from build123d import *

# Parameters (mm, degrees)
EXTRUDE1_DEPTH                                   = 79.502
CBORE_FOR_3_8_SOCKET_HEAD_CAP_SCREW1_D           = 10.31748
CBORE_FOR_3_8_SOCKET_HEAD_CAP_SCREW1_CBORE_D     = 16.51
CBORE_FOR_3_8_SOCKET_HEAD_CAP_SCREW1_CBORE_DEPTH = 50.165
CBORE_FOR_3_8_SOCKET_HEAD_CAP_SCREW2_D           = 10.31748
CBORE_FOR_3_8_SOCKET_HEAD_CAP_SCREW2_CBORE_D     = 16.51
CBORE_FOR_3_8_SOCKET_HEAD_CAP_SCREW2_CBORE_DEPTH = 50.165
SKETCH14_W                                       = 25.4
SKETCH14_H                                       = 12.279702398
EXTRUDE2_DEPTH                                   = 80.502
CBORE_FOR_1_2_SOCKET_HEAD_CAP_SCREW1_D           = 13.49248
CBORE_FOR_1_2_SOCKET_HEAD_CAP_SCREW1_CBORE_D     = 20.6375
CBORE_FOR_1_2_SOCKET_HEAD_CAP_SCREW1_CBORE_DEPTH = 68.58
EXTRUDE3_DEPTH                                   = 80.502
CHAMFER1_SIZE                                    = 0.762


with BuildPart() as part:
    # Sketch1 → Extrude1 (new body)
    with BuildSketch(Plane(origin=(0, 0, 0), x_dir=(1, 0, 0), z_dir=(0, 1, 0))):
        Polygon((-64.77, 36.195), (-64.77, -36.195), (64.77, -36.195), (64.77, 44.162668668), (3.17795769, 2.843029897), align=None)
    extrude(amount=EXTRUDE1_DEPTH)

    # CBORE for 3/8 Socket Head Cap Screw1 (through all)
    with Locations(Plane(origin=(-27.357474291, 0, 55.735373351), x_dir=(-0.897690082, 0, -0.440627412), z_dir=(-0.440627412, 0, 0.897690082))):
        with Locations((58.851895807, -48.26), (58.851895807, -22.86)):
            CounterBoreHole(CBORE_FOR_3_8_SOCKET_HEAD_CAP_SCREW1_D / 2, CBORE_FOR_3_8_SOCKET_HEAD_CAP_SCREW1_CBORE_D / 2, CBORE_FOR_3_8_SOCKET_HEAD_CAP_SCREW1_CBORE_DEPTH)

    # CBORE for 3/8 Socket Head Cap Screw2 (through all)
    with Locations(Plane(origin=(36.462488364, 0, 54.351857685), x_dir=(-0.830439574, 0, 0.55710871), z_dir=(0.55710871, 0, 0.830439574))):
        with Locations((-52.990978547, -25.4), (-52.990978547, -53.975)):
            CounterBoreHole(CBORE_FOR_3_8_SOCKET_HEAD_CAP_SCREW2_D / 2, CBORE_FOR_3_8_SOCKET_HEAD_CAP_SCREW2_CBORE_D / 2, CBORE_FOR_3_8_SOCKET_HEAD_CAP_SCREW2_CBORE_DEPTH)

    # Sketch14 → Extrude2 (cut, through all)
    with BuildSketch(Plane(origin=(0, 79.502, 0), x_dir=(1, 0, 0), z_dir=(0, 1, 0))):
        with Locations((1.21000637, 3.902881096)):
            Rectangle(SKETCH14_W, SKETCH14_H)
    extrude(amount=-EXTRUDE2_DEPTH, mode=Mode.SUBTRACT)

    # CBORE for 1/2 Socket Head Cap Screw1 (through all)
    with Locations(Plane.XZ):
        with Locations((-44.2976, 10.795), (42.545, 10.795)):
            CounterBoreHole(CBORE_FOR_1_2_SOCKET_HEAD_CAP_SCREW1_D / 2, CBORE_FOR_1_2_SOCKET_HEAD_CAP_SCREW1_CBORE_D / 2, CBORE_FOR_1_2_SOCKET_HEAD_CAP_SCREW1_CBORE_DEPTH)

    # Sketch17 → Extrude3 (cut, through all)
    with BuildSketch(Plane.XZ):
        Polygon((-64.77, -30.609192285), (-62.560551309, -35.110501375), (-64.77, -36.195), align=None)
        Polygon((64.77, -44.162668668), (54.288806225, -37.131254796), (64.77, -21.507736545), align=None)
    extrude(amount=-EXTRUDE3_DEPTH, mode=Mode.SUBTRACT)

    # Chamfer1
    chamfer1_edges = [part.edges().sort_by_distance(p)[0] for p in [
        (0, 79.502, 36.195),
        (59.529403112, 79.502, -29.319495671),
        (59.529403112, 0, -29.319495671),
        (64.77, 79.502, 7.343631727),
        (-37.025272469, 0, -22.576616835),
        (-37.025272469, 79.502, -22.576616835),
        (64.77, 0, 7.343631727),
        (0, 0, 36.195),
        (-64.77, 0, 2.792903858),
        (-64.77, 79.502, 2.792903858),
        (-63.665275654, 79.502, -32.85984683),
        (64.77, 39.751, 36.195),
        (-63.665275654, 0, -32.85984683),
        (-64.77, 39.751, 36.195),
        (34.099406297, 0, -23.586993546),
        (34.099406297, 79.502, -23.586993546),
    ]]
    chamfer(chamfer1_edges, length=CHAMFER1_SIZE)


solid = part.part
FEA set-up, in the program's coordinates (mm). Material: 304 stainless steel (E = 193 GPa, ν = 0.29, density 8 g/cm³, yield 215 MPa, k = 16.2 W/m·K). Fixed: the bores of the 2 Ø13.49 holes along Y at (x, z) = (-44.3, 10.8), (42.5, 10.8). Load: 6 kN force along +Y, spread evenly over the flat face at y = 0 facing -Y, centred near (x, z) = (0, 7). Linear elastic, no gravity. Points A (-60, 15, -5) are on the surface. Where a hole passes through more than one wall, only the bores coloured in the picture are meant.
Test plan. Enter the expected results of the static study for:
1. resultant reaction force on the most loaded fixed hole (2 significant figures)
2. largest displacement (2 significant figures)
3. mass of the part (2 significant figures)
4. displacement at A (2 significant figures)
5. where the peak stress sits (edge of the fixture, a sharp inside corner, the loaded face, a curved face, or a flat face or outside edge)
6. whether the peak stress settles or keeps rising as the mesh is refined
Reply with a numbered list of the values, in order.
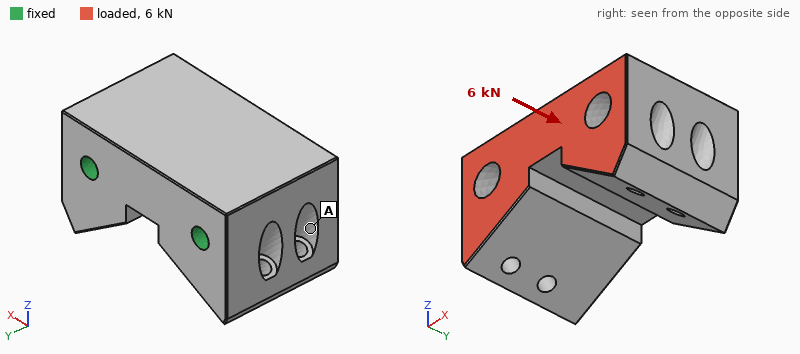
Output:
1. 3.1 kN
2. 3.9 µm
3. 4.0 kg
4. 2.7 µm
5. edge of the fixture
6. keeps rising
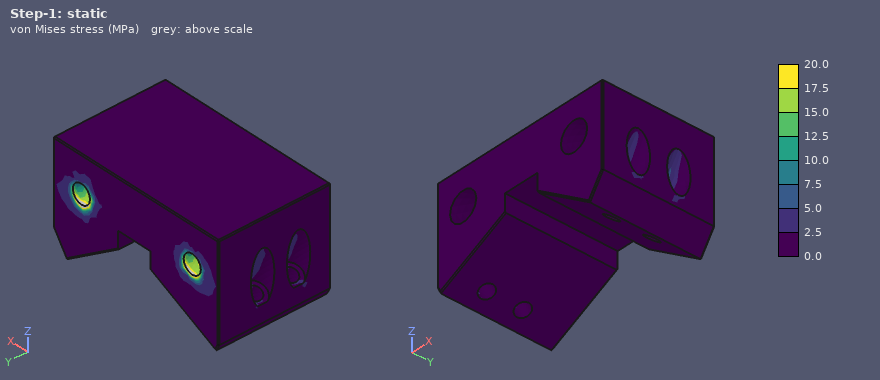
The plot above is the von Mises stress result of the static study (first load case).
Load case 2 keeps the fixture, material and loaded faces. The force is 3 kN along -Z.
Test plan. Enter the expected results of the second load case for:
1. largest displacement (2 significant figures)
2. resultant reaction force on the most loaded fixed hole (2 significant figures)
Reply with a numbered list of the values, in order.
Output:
1. 30 µm
2. 1.5 kN
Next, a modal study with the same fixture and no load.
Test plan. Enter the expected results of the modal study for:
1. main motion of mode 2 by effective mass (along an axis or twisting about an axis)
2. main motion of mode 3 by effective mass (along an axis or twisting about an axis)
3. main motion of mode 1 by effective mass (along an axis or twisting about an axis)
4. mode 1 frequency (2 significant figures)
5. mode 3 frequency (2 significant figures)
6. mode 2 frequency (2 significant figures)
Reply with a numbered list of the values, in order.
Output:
1. along X
2. along X
3. along Z
4. 1400 Hz
5. 4600 Hz
6. 3900 Hz
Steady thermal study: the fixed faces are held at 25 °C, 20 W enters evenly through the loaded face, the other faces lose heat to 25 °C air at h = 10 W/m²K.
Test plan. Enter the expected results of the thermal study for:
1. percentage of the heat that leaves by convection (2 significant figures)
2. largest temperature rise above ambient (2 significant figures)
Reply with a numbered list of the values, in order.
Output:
1. 30 %
2. 19 K
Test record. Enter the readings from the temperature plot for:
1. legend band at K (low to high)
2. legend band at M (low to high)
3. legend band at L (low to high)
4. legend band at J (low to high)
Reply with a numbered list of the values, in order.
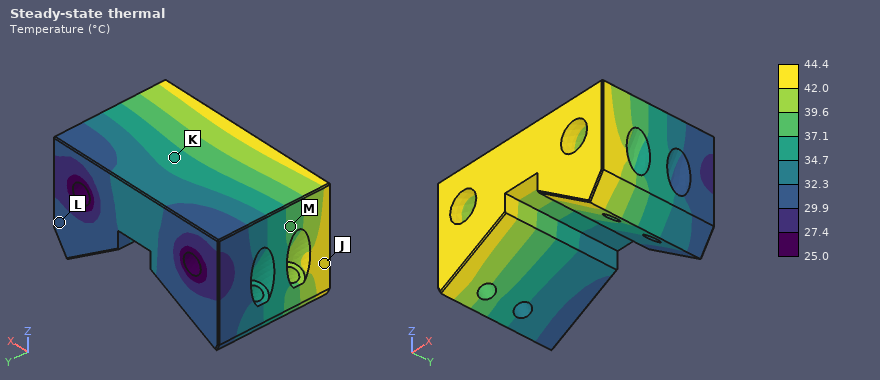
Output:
1. 34.7 to 37.1 °C
2. 37.1 to 39.6 °C
3. 29.9 to 32.3 °C
4. 42.0 to 44.4 °C
